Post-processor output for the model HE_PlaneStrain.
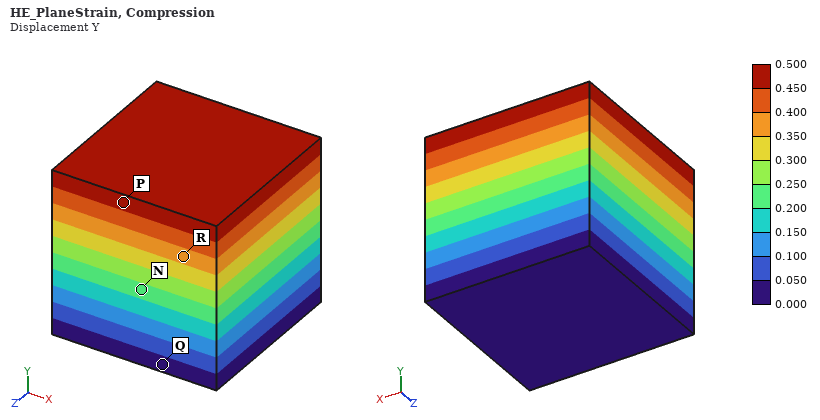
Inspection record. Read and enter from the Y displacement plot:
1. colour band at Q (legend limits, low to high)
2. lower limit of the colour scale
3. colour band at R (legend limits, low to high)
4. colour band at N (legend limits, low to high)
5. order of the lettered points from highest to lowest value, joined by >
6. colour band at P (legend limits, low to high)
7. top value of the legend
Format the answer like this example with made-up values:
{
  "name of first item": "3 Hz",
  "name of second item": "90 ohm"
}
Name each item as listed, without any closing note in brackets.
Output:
{
  "colour band at Q": "0.000 to 0.050",
  "lower limit of the colour scale": "0.000",
  "colour band at R": "0.350 to 0.400",
  "colour band at N": "0.200 to 0.250",
  "order of the lettered points from highest to lowest value, joined by >": "P > R > N > Q",
  "colour band at P": "0.450 to 0.500",
  "top value of the legend": "0.500"
}
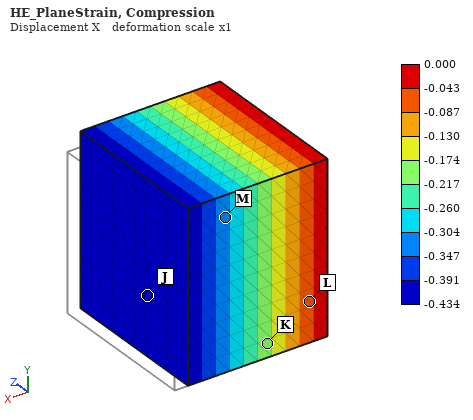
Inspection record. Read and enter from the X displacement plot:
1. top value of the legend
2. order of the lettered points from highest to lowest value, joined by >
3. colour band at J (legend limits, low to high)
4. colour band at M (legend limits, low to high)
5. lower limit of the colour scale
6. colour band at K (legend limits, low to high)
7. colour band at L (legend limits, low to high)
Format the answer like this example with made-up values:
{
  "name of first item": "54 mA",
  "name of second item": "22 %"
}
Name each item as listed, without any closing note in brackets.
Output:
{
  "top value of the legend": "0.000",
  "order of the lettered points from highest to lowest value, joined by >": "L > K > M > J",
  "colour band at J": "-0.434 to -0.391",
  "colour band at M": "-0.347 to -0.304",
  "lower limit of the colour scale": "-0.434",
  "colour band at K": "-0.217 to -0.174",
  "colour band at L": "-0.087 to -0.043"
}
